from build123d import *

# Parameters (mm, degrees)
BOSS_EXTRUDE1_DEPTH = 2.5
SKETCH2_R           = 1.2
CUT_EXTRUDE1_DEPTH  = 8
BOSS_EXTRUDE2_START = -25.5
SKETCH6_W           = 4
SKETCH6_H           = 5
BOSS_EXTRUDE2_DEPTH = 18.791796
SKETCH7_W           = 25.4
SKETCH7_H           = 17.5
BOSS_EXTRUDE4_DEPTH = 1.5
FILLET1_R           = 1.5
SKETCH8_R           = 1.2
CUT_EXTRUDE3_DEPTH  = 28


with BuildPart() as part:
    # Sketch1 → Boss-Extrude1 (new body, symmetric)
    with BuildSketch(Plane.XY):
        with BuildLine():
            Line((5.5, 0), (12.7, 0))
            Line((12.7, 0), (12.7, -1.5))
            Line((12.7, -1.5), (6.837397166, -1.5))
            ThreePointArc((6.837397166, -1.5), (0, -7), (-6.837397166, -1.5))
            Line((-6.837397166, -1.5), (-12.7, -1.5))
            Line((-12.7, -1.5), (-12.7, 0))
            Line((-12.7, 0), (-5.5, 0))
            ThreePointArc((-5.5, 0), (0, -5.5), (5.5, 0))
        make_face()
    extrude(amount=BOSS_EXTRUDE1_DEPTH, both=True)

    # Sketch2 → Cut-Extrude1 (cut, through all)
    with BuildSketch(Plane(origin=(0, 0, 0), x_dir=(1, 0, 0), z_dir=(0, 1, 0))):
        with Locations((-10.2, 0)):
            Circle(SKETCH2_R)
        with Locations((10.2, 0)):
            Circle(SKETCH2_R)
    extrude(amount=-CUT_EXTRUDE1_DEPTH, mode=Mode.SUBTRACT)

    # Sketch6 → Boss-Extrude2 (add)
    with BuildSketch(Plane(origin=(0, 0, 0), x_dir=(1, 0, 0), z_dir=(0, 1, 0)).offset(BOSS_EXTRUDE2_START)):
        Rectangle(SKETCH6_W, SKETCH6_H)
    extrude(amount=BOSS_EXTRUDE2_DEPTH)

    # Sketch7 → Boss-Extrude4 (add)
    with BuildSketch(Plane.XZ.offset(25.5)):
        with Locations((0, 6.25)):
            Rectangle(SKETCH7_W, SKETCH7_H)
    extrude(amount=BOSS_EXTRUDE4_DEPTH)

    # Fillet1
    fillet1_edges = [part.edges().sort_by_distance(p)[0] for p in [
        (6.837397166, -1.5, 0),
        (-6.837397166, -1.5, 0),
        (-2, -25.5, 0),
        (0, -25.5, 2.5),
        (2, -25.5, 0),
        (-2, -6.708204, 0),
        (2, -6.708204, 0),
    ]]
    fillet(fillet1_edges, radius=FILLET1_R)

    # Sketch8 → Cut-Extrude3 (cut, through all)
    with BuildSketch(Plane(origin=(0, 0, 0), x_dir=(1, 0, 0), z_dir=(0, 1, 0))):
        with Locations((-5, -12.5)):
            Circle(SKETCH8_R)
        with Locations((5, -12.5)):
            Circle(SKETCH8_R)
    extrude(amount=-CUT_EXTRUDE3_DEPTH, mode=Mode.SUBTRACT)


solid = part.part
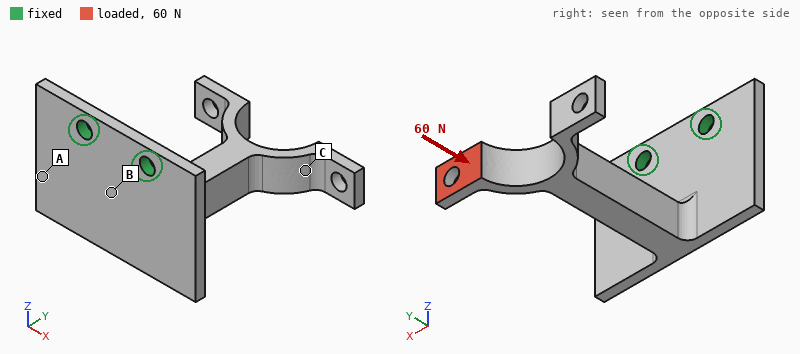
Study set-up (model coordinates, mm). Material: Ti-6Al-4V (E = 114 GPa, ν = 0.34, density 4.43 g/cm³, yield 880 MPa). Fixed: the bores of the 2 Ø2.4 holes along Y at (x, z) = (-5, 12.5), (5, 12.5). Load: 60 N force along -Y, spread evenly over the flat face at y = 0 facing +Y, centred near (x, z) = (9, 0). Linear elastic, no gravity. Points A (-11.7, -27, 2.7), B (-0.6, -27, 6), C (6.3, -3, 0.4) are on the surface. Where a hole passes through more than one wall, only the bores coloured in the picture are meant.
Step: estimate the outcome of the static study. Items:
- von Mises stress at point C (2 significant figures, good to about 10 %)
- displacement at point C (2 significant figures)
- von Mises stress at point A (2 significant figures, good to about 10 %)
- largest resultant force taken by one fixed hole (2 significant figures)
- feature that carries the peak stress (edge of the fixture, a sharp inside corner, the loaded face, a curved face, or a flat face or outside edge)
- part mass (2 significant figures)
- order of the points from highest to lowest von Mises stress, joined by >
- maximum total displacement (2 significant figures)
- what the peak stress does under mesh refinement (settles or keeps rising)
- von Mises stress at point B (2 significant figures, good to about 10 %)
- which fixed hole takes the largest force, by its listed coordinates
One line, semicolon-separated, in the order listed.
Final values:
100 MPa; 0.23 mm; 28 MPa; 74 N; edge of the fixture; 5.6 g; C > B > A; 0.37 mm; keeps rising; 62 MPa; (5, 12.5)
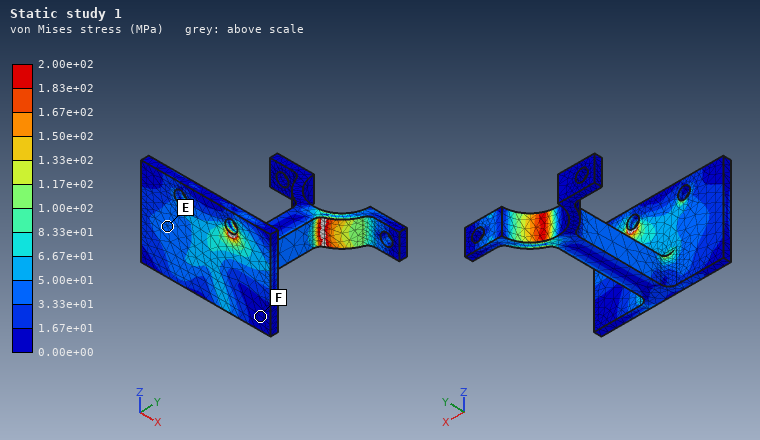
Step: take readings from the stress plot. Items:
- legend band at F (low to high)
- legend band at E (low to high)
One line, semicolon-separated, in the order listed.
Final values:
0.00e+00 to 1.67e+01 MPa; 3.33e+01 to 5.00e+01 MPa
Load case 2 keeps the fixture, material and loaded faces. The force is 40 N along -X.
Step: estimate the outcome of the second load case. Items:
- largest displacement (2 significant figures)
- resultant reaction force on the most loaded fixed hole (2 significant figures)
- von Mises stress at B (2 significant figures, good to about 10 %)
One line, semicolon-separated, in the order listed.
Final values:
0.35 mm; 98 N; 95 MPa
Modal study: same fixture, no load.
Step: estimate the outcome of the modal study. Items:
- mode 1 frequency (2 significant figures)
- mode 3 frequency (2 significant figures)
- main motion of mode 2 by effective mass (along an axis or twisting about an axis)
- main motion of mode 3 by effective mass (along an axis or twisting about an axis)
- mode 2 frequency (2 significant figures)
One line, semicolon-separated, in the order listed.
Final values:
1300 Hz; 5600 Hz; along X; along Y; 1900 Hz
